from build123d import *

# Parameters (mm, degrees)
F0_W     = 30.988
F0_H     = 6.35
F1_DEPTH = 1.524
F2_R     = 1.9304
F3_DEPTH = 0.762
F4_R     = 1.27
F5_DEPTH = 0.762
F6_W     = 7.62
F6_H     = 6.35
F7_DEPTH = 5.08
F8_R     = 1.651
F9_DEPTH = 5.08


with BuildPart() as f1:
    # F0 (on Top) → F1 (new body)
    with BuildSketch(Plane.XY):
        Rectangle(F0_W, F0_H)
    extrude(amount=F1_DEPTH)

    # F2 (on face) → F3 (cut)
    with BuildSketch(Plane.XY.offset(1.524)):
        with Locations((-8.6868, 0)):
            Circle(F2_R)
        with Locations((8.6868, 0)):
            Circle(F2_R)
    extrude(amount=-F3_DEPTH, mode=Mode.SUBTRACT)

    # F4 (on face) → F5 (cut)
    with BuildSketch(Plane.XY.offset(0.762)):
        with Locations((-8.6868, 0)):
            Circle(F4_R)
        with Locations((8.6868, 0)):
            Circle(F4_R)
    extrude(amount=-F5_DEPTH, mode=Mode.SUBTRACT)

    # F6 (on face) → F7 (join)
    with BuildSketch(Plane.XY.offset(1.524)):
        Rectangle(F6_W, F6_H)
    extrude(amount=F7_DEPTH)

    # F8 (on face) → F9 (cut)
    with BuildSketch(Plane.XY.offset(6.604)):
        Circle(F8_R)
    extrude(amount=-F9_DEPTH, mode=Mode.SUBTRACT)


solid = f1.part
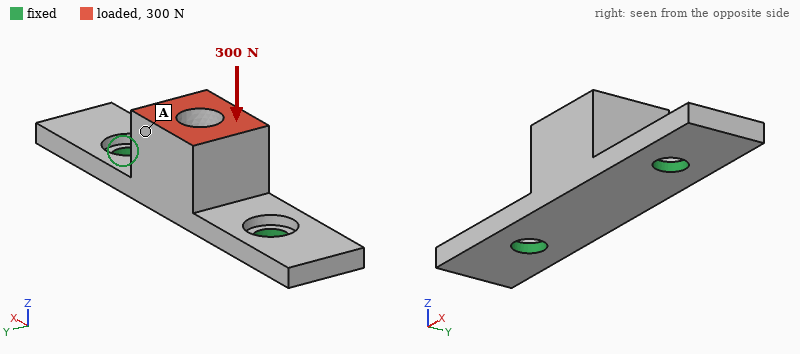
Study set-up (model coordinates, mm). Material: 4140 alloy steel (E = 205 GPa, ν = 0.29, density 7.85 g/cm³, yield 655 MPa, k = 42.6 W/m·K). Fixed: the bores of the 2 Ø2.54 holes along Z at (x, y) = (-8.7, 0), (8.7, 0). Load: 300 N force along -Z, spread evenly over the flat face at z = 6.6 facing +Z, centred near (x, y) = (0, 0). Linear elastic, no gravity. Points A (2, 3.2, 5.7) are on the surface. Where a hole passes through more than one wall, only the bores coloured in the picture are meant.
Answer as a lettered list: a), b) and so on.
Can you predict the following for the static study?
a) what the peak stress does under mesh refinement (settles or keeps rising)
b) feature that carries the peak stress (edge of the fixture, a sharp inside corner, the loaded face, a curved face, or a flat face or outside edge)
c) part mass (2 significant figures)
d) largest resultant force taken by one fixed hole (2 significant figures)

a) keeps rising
b) edge of the fixture
c) 3.7 g
d) 240 N
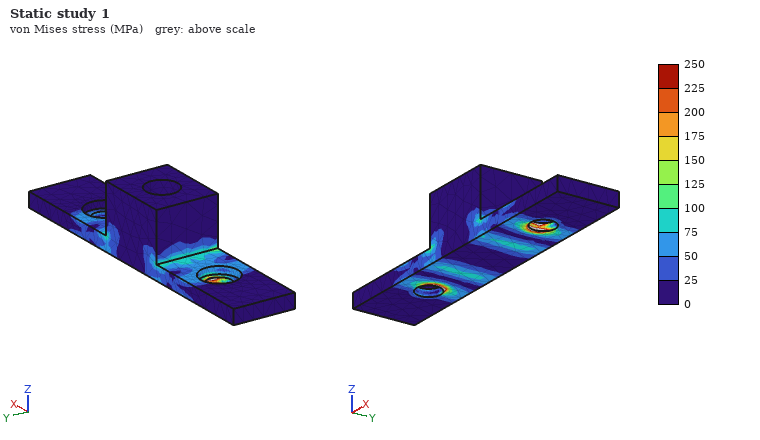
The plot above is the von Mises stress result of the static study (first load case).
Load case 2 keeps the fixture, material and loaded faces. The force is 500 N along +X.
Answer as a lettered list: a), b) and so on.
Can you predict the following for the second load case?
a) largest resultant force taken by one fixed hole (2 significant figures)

a) 340 N
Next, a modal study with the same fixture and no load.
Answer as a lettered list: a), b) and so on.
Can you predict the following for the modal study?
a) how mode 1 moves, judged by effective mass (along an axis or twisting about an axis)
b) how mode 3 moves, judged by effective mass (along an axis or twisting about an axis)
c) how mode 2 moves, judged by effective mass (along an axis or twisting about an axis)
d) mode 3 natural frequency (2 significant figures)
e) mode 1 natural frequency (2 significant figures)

a) along Y
b) twisting about Y
c) along Z
d) 23 kHz
e) 12 kHz
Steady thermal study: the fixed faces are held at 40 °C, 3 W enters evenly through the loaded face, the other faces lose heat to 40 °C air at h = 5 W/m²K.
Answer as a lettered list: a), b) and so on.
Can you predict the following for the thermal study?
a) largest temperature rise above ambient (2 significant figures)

a) 31 K
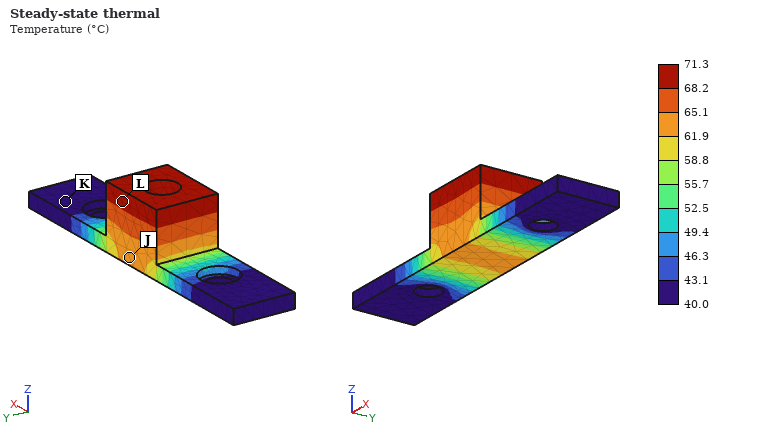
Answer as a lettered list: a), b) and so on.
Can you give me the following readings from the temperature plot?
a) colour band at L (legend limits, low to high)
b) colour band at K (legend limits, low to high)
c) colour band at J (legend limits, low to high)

a) 68.2 to 71.3 °C
b) 40.0 to 43.1 °C
c) 61.9 to 65.1 °C
